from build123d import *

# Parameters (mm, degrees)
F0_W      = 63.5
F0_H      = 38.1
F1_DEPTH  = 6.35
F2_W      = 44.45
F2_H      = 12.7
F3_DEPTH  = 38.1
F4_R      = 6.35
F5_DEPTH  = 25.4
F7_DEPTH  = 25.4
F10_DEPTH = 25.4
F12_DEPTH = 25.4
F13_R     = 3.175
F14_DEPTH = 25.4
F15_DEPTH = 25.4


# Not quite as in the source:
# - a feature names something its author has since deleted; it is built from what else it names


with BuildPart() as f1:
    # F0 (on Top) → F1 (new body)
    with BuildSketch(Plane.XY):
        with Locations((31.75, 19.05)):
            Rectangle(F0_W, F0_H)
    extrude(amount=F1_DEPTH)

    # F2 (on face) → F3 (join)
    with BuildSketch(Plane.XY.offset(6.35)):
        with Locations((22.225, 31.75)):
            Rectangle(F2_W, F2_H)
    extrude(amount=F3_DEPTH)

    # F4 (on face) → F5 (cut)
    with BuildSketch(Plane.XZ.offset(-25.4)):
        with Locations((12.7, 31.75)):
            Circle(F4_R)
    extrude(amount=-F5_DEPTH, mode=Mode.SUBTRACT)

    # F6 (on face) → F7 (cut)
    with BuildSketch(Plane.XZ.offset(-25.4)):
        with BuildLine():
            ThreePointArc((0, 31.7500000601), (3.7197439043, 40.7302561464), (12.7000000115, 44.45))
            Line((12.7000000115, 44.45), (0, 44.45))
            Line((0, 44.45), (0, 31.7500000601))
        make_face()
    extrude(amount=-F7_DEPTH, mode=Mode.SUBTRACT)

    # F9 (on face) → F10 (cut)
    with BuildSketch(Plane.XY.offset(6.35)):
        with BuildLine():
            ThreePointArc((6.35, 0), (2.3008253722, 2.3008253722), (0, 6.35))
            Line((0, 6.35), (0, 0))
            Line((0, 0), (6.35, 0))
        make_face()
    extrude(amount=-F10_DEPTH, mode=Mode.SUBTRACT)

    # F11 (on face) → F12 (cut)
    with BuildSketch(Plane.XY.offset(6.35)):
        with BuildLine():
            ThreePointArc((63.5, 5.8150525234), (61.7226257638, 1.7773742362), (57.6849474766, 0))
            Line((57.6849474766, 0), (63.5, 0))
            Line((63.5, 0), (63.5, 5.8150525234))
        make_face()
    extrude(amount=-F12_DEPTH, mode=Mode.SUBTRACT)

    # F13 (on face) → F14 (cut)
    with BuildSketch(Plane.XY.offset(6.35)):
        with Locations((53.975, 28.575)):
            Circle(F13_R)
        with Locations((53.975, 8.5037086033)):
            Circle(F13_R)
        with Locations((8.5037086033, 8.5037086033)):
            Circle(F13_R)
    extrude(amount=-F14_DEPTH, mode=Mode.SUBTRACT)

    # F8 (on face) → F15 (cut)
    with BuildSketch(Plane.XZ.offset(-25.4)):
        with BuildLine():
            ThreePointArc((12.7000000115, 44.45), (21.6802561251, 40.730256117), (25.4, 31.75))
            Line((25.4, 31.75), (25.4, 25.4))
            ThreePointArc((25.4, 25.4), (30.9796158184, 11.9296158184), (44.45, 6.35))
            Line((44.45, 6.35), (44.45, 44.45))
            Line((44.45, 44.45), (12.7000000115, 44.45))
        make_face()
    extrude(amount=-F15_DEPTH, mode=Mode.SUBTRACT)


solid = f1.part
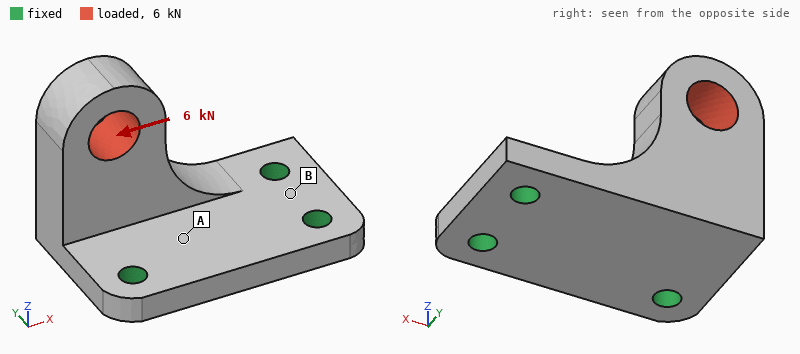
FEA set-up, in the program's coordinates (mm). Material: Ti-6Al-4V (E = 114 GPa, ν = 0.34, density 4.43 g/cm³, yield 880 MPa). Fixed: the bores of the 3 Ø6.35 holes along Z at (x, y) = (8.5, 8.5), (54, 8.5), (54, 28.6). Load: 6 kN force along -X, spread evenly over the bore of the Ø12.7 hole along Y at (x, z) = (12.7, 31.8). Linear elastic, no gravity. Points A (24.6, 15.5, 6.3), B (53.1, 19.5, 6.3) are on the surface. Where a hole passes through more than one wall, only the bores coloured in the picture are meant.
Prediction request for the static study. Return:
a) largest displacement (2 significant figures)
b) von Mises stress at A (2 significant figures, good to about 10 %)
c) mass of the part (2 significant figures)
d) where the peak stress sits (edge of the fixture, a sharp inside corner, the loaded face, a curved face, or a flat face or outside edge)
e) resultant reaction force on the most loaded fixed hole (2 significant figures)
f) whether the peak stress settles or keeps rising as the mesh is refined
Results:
0.37 mm
110 MPa
110 g
edge of the fixture
4.6 kN
keeps rising
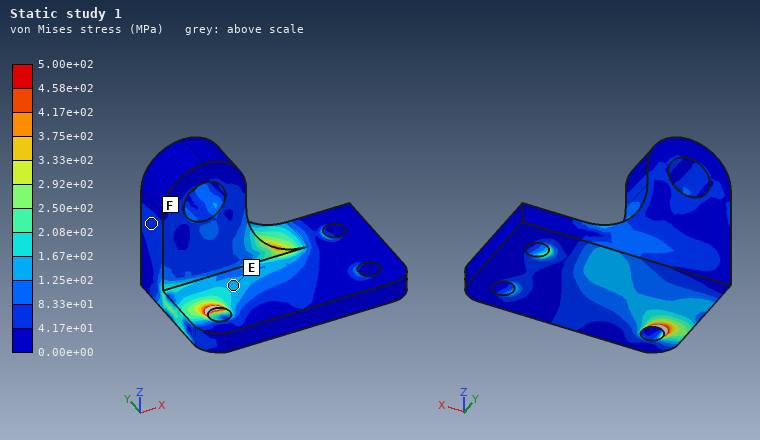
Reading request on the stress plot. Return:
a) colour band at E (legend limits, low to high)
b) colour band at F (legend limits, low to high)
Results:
1.25e+02 to 1.67e+02 MPa
4.17e+01 to 8.33e+01 MPa
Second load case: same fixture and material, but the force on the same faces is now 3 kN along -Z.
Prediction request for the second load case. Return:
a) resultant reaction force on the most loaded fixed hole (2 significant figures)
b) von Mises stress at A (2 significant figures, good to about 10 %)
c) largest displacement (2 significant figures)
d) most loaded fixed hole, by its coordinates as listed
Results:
2.4 kN
58 MPa
0.22 mm
(8.5, 8.5)
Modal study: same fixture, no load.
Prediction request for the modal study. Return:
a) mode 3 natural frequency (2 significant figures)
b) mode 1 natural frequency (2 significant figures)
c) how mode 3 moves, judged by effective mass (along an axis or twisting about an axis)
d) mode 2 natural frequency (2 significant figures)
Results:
8000 Hz
2400 Hz
along Z
5500 Hz
